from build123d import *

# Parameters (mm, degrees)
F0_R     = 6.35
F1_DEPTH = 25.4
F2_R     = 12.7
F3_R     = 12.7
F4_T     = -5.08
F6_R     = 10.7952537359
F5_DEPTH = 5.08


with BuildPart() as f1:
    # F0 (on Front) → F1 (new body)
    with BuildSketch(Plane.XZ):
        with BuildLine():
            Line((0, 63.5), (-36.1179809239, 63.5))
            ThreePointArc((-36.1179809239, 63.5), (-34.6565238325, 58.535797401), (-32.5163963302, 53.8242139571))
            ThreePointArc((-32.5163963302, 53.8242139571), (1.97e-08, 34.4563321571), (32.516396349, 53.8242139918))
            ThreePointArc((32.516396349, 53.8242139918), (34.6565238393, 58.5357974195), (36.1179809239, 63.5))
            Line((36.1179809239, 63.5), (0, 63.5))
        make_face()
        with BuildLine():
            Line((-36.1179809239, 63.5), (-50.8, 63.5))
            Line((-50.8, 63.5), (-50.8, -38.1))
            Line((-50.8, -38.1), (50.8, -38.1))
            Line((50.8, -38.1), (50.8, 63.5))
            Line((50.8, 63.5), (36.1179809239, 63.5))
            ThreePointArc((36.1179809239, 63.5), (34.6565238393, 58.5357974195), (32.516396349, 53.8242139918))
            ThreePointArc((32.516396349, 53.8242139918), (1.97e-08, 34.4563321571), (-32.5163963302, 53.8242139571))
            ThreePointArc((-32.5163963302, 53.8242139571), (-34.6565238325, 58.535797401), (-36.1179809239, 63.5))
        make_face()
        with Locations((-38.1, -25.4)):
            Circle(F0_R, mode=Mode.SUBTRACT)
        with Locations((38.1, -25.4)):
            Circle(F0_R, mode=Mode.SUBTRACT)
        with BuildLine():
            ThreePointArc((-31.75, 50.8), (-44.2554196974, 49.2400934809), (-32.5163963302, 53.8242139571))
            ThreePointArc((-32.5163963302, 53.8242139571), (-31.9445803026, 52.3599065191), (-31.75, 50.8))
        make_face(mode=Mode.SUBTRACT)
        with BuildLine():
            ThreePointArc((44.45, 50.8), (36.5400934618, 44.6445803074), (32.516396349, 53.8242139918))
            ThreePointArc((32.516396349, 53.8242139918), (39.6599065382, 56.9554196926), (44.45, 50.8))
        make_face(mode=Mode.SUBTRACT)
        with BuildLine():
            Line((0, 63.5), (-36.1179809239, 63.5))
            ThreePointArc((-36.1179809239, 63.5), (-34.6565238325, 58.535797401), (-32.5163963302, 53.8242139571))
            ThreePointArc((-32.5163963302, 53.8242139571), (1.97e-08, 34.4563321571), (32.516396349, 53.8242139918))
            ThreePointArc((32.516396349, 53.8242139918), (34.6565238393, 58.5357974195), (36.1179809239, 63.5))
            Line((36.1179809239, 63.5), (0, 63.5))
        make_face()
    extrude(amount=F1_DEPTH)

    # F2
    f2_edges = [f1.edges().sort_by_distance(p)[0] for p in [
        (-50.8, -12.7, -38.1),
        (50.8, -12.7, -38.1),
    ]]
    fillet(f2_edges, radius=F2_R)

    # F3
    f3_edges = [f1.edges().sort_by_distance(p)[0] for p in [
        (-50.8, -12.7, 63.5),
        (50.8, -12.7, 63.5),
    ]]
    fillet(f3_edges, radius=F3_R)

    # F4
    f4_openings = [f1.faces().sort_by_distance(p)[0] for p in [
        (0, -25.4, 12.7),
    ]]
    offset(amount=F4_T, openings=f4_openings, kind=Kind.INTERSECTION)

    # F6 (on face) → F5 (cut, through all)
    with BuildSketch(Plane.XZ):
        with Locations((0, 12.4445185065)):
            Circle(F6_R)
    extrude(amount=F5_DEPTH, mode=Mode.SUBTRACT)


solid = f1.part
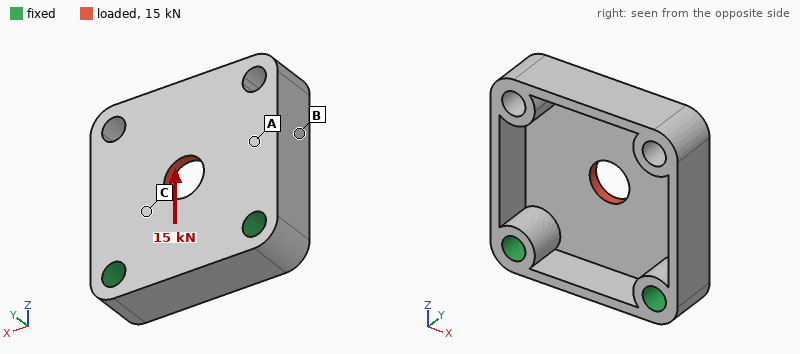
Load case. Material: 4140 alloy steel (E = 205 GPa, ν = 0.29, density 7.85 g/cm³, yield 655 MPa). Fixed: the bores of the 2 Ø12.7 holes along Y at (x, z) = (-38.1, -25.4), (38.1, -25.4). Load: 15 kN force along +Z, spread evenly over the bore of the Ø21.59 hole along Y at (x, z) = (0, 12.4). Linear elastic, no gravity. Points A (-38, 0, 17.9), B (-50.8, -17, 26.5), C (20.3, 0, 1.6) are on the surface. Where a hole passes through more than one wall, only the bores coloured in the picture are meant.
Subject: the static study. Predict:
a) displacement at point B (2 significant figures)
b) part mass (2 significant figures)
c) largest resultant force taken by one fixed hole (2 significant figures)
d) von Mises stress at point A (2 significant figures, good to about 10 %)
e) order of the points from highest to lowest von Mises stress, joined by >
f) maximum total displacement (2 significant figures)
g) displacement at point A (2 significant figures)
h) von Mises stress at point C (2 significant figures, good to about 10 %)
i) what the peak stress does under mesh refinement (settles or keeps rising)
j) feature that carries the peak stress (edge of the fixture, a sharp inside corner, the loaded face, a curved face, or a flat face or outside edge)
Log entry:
8.6 µm
790 g
7.8 kN
18 MPa
C > A > B
21 µm
7.9 µm
37 MPa
keeps rising
edge of the fixture
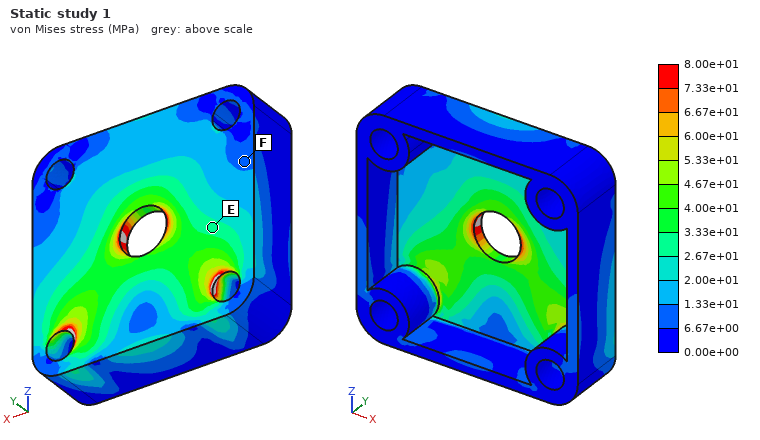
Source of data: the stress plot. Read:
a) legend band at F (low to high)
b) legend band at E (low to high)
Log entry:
6.67e+00 to 1.33e+01 MPa
2.67e+01 to 3.33e+01 MPa
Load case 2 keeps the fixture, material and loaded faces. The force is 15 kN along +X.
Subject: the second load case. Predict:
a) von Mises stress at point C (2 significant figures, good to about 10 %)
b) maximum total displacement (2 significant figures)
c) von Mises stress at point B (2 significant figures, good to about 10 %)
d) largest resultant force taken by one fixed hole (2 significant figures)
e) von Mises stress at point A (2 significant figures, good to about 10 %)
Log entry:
52 MPa
37 µm
8.7 MPa
9.7 kN
15 MPa
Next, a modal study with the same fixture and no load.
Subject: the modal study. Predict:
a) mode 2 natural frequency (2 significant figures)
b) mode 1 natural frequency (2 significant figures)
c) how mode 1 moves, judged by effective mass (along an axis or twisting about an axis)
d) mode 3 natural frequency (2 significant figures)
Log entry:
2200 Hz
1500 Hz
along Y
4800 Hz
